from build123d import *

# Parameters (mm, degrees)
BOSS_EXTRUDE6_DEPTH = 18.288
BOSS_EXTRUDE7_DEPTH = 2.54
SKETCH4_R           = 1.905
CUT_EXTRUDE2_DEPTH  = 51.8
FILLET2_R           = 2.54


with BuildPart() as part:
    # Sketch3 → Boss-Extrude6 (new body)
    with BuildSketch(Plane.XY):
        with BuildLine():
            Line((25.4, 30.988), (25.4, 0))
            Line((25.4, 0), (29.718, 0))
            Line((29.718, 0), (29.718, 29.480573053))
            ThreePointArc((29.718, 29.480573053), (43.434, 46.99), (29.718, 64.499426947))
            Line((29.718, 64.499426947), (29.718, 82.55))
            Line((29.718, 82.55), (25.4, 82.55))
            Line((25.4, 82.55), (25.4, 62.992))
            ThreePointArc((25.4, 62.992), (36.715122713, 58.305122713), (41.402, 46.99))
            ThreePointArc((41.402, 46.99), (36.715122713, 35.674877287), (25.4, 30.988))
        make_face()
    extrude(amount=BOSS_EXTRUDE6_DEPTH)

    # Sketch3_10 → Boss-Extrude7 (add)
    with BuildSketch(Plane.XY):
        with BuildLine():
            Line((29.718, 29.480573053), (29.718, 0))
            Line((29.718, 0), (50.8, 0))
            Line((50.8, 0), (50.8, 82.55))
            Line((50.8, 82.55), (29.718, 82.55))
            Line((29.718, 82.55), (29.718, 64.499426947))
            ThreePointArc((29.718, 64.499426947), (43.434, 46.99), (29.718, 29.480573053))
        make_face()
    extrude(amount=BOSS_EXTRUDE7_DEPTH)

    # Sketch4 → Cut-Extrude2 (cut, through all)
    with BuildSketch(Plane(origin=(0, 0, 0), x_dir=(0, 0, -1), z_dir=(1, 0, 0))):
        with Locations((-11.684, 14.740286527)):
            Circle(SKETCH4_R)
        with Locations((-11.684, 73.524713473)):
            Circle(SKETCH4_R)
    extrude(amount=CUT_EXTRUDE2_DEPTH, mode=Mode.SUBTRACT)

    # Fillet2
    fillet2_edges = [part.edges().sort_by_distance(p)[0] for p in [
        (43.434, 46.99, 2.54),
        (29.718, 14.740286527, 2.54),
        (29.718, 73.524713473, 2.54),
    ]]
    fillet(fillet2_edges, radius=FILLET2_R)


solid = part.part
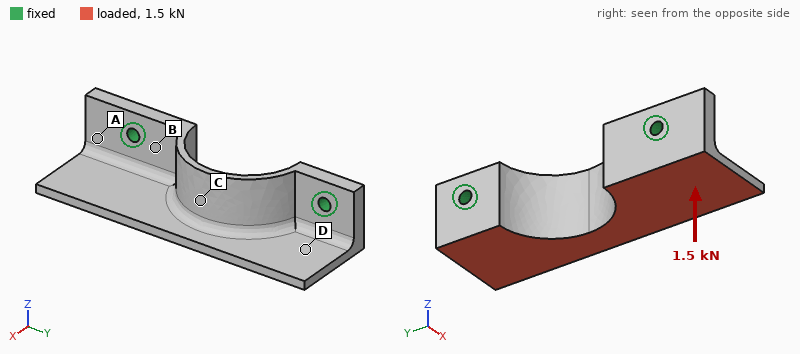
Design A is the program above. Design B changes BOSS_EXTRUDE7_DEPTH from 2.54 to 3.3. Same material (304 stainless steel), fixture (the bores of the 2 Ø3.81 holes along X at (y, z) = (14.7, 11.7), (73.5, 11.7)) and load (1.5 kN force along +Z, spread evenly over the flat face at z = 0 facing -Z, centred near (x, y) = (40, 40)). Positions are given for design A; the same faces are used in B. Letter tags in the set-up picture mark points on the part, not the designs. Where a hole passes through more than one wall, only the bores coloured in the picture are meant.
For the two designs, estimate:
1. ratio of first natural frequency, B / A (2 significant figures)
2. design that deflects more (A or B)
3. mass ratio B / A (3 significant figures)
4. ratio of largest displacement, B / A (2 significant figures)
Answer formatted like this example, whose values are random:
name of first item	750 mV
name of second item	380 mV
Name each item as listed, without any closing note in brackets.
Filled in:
ratio of first natural frequency, B / A	0.97
design that deflects more	A
mass ratio B / A	1.11
ratio of largest displacement, B / A	0.72
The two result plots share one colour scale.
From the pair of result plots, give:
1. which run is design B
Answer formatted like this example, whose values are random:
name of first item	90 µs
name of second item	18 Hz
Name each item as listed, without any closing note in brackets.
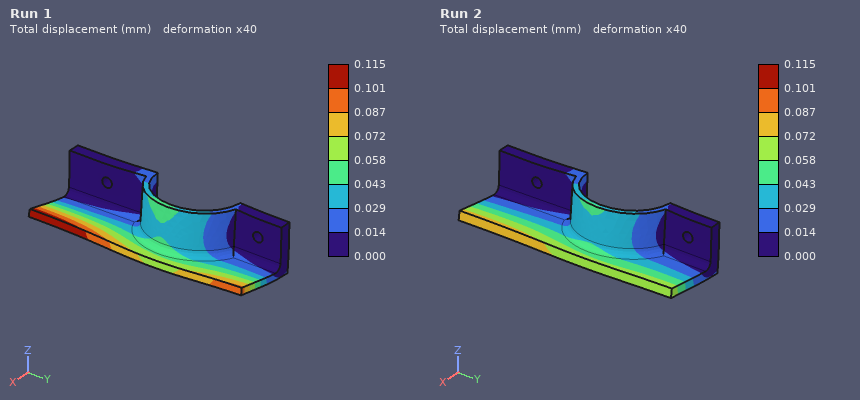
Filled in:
which run is design B	Run 2
